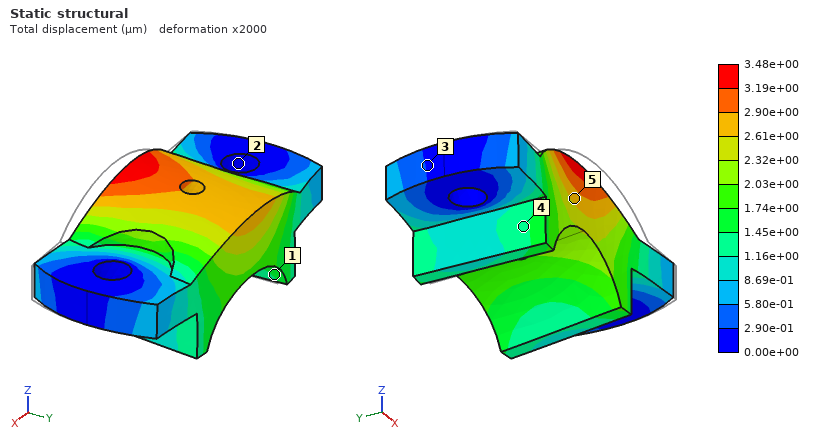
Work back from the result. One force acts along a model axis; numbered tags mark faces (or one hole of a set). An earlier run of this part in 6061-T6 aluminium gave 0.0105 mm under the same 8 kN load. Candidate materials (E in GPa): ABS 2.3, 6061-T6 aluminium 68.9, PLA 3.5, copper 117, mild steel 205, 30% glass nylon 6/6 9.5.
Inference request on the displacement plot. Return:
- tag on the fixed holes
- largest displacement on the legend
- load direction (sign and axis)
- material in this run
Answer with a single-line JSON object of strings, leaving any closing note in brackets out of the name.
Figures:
{"tag on the fixed holes": "2", "largest displacement on the legend": "3.48e+00 µm", "load direction": "+Y", "material in this run": "mild steel"}
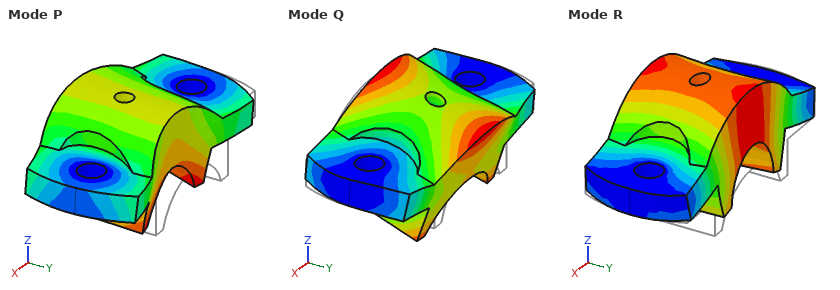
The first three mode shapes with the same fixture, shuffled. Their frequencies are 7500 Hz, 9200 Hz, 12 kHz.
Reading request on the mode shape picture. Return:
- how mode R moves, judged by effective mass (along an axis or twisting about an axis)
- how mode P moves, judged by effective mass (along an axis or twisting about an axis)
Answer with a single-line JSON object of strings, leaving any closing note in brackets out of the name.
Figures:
{"how mode R moves, judged by effective mass": "along Z", "how mode P moves, judged by effective mass": "along Y"}
